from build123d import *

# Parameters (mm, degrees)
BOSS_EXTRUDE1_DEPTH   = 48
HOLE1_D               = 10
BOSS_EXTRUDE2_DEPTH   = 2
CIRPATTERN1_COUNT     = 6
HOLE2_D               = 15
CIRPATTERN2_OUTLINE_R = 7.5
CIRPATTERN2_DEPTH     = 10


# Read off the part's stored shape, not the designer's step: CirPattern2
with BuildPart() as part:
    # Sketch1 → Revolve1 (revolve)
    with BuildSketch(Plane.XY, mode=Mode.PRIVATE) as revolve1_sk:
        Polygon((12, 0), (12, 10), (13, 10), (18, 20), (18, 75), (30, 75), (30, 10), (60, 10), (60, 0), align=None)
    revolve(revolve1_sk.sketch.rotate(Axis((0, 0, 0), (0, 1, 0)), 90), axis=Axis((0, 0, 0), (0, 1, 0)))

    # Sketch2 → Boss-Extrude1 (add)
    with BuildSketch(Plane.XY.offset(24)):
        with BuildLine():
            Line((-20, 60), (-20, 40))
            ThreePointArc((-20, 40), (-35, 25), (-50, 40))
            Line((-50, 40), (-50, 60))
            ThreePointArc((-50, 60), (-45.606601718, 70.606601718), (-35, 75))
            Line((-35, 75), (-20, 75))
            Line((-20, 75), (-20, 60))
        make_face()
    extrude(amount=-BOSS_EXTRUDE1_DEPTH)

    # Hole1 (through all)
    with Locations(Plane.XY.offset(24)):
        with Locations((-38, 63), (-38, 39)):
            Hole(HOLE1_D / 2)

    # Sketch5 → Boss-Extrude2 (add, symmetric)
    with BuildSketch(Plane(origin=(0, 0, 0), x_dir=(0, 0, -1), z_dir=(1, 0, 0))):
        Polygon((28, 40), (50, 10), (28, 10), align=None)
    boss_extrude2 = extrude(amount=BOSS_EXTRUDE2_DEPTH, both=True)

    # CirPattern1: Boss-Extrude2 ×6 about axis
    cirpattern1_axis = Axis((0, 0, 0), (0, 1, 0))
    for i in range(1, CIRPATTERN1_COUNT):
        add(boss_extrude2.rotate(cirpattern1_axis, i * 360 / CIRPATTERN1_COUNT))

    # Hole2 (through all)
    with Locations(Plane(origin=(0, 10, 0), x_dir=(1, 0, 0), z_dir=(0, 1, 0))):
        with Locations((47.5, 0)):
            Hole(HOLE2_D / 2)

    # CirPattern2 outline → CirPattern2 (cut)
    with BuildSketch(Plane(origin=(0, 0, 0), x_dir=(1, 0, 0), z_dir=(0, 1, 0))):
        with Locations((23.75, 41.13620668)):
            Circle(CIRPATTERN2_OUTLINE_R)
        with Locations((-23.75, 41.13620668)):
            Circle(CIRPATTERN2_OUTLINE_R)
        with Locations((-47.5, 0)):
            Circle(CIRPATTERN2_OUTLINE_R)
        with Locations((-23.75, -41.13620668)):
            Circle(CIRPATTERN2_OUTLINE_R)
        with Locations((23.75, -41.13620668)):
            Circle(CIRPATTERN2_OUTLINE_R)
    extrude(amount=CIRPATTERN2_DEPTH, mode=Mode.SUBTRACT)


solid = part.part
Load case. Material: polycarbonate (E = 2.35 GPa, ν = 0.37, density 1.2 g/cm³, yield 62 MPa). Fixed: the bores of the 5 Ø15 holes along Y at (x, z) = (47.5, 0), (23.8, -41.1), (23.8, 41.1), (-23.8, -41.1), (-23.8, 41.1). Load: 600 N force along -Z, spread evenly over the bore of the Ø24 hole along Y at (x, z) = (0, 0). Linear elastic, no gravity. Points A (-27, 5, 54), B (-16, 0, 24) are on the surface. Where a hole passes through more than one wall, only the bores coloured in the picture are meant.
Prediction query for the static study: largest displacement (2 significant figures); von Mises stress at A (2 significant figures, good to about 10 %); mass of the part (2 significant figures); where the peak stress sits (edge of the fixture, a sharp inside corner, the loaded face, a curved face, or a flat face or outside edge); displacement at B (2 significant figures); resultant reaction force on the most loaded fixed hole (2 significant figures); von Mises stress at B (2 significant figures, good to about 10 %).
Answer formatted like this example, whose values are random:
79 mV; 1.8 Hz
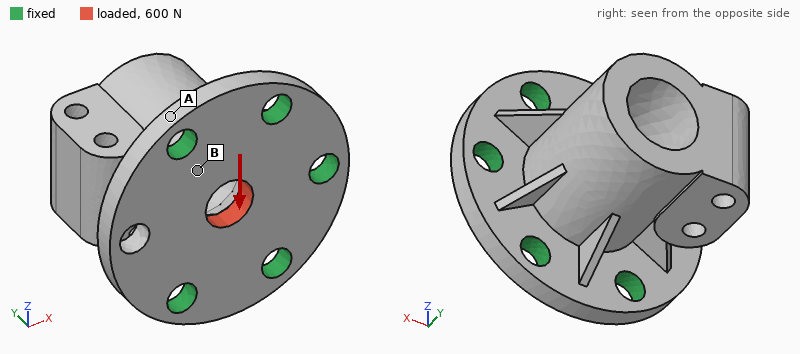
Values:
9.3 µm; 0.13 MPa; 320 g; a flat face or outside edge; 3.0 µm; 160 N; 0.62 MPa
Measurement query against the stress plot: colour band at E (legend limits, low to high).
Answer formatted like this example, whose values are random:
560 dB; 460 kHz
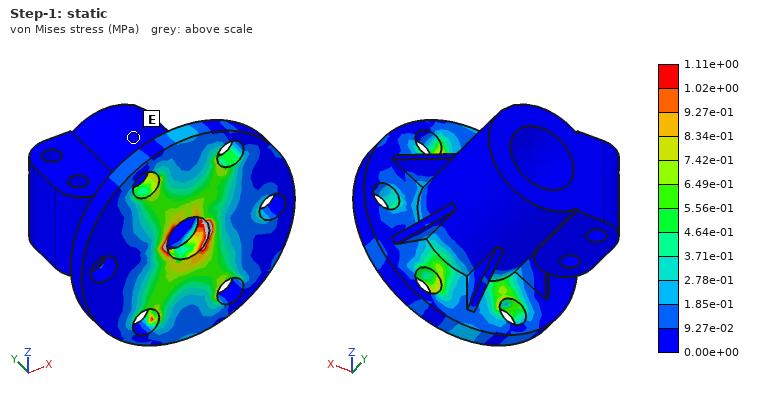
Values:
0.00e+00 to 9.27e-02 MPa
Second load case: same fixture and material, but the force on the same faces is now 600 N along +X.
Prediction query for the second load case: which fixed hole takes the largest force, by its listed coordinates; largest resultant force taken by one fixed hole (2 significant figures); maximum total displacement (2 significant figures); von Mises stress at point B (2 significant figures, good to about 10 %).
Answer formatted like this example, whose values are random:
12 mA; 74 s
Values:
(47.5, 0); 180 N; 15 µm; 0.52 MPa
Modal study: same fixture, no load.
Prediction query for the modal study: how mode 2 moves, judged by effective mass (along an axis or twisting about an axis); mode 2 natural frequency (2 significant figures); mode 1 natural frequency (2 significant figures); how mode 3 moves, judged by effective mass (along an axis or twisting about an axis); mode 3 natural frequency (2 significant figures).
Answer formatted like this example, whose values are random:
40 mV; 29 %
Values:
along Z; 1200 Hz; 930 Hz; along Y; 2000 Hz
